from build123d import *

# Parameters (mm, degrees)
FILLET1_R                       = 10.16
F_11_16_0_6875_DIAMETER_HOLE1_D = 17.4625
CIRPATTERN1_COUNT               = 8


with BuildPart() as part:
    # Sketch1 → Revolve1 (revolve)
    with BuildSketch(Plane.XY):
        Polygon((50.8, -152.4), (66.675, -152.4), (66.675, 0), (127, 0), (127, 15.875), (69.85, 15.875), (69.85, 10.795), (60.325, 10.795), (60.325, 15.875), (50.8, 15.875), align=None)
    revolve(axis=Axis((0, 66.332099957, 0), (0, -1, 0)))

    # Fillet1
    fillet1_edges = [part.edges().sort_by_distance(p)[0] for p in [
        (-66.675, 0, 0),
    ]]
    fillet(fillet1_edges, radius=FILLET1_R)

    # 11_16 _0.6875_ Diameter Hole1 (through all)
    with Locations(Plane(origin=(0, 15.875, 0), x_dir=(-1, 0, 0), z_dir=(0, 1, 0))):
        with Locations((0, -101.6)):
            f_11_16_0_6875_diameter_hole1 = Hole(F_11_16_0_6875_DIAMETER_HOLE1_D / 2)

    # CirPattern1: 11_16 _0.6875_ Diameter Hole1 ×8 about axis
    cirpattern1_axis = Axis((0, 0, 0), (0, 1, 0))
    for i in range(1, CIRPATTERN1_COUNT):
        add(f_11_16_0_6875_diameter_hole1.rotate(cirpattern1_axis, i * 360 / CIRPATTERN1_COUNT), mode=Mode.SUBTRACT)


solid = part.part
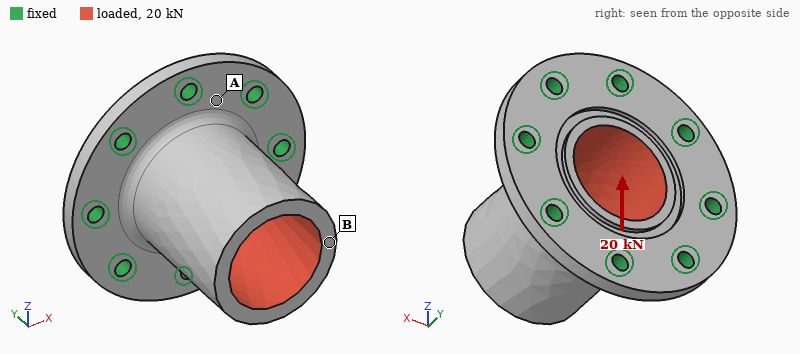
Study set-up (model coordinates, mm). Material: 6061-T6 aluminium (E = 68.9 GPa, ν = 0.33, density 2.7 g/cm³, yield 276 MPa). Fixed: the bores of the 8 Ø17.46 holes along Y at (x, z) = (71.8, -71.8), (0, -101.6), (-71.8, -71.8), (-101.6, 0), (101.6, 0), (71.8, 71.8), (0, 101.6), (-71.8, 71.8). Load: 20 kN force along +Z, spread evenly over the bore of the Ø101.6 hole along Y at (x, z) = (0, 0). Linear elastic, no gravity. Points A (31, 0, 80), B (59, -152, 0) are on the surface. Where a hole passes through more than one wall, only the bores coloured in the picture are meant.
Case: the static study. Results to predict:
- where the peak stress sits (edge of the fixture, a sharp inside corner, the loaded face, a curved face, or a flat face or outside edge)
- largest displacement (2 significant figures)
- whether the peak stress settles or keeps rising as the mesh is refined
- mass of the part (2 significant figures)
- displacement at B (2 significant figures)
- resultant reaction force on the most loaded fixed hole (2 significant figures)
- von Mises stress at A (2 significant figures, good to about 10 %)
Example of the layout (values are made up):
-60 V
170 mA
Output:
edge of the fixture
80 µm
keeps rising
4.1 kg
74 µm
6.3 kN
7.5 MPa
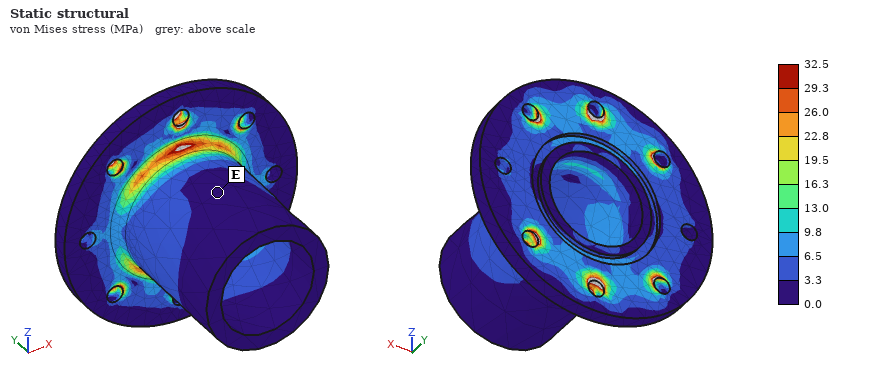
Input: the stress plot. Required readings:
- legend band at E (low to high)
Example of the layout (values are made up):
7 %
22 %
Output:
0.0 to 3.3 MPa
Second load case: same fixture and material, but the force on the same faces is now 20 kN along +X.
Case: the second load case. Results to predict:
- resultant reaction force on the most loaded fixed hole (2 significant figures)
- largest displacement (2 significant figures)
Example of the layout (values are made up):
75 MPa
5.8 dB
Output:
6.3 kN
80 µm
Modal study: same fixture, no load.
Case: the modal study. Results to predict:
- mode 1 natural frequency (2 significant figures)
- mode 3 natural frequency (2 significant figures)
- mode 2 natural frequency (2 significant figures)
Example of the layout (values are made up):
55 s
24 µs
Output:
1800 Hz
3200 Hz
1800 Hz
